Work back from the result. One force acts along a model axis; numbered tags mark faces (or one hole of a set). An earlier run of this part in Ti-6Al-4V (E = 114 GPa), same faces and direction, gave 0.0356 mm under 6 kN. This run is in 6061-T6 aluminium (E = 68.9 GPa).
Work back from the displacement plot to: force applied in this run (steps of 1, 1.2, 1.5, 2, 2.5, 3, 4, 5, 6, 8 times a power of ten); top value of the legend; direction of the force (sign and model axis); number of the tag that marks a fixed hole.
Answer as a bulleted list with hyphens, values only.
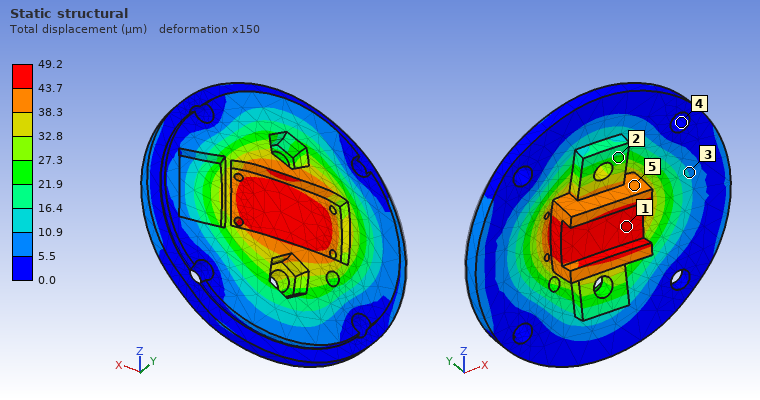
- 5 kN
- 49.2 µm
- +Y
- 4
